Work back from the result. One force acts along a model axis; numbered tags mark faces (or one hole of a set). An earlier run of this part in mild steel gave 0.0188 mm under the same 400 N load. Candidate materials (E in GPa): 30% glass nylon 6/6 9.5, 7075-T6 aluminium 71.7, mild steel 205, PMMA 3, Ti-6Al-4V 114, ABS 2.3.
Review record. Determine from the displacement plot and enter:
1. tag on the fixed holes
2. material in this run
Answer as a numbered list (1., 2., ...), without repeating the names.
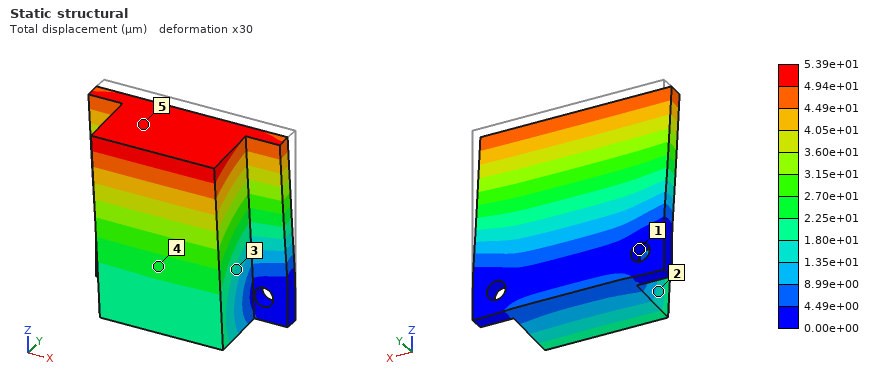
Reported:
1. 1
2. 7075-T6 aluminium
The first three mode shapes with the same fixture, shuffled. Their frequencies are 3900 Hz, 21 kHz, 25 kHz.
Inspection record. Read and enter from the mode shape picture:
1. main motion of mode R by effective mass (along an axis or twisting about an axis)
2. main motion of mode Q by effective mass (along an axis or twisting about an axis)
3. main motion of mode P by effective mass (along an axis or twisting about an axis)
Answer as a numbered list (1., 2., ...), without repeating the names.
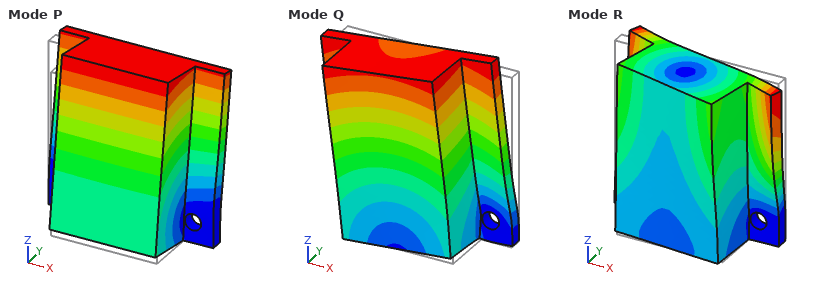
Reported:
1. twisting about Z
2. along X
3. along Y
